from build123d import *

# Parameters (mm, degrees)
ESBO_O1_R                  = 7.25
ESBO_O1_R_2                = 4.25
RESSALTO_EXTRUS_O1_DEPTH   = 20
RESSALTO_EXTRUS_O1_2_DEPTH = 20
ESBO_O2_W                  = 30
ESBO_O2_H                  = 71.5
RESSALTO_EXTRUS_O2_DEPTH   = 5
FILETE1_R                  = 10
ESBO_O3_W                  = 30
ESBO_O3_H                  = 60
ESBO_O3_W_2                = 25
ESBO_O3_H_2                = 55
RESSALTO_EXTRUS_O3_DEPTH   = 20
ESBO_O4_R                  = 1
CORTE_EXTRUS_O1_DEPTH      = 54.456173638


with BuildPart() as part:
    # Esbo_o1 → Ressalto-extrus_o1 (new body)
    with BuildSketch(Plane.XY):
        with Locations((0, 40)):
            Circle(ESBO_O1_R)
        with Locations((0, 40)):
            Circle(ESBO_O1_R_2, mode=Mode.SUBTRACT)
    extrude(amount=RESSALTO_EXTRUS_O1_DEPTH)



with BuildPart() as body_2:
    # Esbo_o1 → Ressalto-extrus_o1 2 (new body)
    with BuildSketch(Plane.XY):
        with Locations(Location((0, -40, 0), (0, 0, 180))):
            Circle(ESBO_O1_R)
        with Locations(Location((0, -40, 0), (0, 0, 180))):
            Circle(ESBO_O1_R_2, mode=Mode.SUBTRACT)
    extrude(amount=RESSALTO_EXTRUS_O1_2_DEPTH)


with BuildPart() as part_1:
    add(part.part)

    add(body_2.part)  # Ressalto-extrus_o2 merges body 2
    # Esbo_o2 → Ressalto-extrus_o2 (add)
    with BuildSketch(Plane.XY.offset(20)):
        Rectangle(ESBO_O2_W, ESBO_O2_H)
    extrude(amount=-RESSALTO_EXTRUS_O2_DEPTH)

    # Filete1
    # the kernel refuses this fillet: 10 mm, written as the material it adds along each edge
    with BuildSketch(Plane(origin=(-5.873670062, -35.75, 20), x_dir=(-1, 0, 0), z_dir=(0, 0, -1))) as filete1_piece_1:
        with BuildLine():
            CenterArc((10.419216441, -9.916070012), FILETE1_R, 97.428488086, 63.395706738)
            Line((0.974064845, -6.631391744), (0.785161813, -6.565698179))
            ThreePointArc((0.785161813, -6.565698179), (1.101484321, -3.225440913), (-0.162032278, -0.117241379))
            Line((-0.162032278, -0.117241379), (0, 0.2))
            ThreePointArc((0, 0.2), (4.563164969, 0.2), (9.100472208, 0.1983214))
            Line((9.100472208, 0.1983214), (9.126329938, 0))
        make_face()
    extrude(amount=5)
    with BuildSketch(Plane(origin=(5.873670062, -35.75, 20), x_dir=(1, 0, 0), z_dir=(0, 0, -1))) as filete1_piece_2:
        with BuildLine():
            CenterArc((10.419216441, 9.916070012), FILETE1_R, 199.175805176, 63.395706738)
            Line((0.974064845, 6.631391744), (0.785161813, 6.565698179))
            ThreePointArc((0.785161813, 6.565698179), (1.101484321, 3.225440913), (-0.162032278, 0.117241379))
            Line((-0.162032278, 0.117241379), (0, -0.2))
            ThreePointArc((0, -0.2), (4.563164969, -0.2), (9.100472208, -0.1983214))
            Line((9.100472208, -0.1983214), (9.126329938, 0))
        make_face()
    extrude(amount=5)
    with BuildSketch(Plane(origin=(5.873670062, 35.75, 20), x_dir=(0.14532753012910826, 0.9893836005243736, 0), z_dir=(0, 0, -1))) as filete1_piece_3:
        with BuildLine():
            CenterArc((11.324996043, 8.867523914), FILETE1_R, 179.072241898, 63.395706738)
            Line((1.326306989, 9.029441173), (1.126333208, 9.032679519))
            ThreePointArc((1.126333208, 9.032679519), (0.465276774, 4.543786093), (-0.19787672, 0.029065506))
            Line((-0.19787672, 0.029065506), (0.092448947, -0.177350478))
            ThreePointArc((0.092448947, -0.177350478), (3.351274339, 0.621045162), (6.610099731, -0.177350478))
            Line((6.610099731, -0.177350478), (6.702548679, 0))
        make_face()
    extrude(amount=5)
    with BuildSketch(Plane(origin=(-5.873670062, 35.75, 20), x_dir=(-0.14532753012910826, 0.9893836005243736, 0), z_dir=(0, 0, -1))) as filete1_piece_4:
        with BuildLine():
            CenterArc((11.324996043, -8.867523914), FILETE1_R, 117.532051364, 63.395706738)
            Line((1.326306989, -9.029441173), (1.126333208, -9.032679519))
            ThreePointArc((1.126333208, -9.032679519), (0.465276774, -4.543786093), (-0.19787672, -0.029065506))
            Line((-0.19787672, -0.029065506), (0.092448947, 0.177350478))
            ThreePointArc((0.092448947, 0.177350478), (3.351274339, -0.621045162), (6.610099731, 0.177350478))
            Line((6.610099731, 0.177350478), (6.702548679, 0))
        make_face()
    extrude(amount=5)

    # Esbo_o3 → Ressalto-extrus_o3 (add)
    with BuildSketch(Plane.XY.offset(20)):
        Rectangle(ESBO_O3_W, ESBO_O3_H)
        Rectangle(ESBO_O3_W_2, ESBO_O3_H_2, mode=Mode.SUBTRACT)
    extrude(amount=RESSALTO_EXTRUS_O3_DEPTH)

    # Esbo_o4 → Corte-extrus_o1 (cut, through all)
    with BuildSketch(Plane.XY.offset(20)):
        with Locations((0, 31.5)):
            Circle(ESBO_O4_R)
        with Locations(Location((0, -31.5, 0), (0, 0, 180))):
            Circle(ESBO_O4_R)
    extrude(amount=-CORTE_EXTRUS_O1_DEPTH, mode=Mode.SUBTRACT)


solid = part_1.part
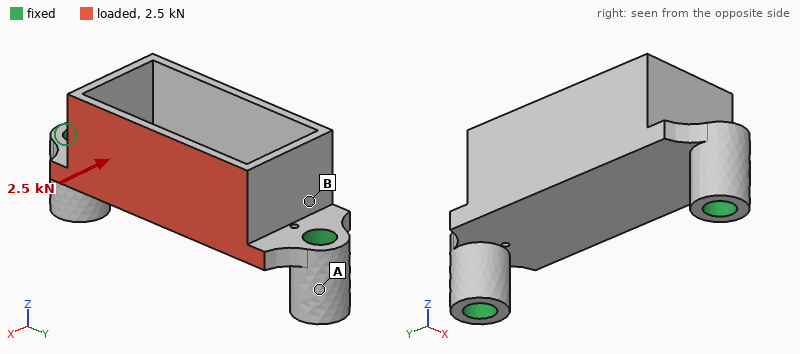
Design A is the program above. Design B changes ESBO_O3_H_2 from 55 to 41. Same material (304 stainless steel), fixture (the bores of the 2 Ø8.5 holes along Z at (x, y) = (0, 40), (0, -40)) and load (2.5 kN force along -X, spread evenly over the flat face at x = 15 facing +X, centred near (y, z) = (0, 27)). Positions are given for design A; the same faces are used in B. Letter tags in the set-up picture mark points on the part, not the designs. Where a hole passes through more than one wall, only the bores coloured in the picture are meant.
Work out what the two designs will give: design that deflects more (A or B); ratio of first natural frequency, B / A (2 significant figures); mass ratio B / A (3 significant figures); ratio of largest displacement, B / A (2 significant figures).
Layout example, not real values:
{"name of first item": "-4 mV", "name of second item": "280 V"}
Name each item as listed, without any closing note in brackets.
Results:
{"design that deflects more": "A", "ratio of first natural frequency, B / A": "0.95", "mass ratio B / A": "1.30", "ratio of largest displacement, B / A": "0.55"}
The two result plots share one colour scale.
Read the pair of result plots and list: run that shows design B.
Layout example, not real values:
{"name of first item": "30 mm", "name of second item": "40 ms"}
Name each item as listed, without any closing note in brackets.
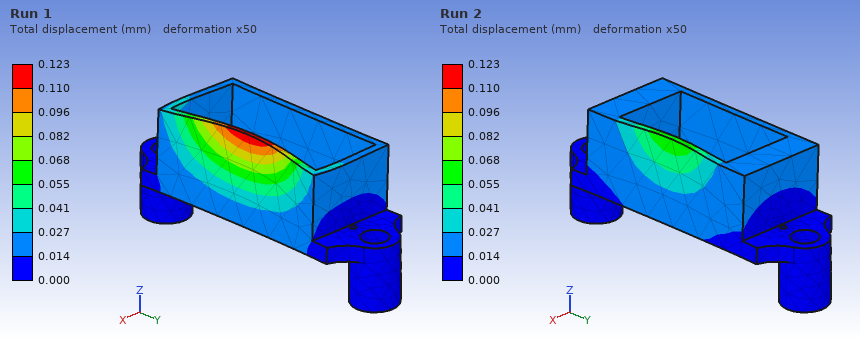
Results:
{"run that shows design B": "Run 2"}
